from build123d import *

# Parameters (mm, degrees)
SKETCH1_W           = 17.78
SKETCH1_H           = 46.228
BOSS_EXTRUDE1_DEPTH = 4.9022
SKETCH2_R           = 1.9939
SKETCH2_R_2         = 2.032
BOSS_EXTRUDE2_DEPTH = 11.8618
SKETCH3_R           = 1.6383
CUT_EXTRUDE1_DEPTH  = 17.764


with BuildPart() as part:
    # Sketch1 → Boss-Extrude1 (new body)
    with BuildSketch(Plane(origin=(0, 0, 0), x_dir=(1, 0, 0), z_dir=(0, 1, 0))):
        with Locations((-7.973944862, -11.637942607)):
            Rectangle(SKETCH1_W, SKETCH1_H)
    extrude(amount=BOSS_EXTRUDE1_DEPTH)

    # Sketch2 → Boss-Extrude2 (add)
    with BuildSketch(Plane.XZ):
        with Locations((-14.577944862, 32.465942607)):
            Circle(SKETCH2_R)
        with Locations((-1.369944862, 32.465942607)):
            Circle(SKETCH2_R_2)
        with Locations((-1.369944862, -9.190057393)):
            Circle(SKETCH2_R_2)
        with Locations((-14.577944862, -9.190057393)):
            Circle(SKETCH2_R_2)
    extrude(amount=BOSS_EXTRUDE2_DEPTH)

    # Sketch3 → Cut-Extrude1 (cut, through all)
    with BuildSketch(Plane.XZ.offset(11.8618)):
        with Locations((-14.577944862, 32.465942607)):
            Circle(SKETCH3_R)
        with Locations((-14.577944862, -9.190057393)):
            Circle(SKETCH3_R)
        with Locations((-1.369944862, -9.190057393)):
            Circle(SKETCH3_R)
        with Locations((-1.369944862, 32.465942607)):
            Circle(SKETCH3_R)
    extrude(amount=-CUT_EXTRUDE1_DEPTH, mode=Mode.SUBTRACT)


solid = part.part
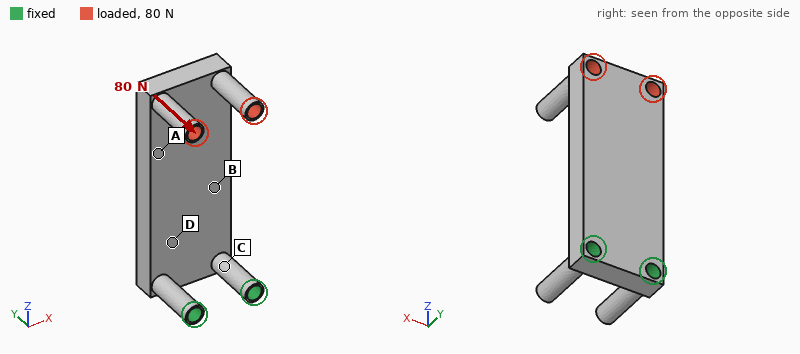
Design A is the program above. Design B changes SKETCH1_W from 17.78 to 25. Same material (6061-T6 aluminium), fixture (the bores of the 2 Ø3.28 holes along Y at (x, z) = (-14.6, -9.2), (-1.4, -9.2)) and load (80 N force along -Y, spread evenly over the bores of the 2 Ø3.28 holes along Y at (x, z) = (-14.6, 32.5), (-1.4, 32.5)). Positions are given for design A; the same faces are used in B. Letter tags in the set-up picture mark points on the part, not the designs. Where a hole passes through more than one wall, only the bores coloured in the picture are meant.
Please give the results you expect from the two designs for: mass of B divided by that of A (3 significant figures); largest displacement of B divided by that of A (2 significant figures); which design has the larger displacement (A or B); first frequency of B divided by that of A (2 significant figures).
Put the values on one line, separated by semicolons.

1.40; 0.72; A; 1.00
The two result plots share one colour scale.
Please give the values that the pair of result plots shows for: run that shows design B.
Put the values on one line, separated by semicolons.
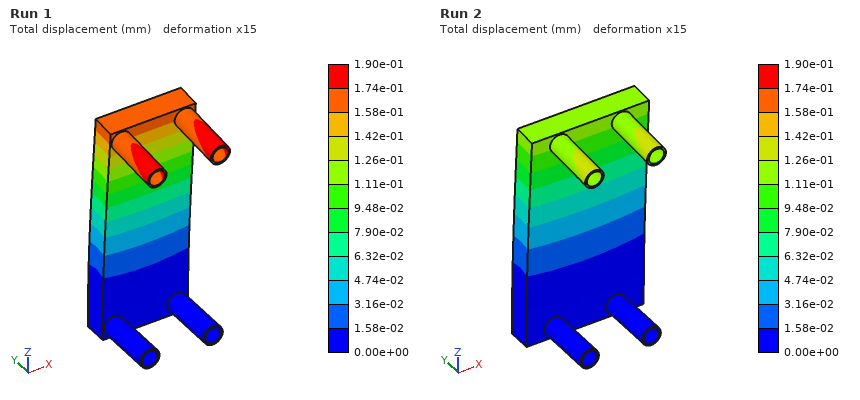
Run 2
